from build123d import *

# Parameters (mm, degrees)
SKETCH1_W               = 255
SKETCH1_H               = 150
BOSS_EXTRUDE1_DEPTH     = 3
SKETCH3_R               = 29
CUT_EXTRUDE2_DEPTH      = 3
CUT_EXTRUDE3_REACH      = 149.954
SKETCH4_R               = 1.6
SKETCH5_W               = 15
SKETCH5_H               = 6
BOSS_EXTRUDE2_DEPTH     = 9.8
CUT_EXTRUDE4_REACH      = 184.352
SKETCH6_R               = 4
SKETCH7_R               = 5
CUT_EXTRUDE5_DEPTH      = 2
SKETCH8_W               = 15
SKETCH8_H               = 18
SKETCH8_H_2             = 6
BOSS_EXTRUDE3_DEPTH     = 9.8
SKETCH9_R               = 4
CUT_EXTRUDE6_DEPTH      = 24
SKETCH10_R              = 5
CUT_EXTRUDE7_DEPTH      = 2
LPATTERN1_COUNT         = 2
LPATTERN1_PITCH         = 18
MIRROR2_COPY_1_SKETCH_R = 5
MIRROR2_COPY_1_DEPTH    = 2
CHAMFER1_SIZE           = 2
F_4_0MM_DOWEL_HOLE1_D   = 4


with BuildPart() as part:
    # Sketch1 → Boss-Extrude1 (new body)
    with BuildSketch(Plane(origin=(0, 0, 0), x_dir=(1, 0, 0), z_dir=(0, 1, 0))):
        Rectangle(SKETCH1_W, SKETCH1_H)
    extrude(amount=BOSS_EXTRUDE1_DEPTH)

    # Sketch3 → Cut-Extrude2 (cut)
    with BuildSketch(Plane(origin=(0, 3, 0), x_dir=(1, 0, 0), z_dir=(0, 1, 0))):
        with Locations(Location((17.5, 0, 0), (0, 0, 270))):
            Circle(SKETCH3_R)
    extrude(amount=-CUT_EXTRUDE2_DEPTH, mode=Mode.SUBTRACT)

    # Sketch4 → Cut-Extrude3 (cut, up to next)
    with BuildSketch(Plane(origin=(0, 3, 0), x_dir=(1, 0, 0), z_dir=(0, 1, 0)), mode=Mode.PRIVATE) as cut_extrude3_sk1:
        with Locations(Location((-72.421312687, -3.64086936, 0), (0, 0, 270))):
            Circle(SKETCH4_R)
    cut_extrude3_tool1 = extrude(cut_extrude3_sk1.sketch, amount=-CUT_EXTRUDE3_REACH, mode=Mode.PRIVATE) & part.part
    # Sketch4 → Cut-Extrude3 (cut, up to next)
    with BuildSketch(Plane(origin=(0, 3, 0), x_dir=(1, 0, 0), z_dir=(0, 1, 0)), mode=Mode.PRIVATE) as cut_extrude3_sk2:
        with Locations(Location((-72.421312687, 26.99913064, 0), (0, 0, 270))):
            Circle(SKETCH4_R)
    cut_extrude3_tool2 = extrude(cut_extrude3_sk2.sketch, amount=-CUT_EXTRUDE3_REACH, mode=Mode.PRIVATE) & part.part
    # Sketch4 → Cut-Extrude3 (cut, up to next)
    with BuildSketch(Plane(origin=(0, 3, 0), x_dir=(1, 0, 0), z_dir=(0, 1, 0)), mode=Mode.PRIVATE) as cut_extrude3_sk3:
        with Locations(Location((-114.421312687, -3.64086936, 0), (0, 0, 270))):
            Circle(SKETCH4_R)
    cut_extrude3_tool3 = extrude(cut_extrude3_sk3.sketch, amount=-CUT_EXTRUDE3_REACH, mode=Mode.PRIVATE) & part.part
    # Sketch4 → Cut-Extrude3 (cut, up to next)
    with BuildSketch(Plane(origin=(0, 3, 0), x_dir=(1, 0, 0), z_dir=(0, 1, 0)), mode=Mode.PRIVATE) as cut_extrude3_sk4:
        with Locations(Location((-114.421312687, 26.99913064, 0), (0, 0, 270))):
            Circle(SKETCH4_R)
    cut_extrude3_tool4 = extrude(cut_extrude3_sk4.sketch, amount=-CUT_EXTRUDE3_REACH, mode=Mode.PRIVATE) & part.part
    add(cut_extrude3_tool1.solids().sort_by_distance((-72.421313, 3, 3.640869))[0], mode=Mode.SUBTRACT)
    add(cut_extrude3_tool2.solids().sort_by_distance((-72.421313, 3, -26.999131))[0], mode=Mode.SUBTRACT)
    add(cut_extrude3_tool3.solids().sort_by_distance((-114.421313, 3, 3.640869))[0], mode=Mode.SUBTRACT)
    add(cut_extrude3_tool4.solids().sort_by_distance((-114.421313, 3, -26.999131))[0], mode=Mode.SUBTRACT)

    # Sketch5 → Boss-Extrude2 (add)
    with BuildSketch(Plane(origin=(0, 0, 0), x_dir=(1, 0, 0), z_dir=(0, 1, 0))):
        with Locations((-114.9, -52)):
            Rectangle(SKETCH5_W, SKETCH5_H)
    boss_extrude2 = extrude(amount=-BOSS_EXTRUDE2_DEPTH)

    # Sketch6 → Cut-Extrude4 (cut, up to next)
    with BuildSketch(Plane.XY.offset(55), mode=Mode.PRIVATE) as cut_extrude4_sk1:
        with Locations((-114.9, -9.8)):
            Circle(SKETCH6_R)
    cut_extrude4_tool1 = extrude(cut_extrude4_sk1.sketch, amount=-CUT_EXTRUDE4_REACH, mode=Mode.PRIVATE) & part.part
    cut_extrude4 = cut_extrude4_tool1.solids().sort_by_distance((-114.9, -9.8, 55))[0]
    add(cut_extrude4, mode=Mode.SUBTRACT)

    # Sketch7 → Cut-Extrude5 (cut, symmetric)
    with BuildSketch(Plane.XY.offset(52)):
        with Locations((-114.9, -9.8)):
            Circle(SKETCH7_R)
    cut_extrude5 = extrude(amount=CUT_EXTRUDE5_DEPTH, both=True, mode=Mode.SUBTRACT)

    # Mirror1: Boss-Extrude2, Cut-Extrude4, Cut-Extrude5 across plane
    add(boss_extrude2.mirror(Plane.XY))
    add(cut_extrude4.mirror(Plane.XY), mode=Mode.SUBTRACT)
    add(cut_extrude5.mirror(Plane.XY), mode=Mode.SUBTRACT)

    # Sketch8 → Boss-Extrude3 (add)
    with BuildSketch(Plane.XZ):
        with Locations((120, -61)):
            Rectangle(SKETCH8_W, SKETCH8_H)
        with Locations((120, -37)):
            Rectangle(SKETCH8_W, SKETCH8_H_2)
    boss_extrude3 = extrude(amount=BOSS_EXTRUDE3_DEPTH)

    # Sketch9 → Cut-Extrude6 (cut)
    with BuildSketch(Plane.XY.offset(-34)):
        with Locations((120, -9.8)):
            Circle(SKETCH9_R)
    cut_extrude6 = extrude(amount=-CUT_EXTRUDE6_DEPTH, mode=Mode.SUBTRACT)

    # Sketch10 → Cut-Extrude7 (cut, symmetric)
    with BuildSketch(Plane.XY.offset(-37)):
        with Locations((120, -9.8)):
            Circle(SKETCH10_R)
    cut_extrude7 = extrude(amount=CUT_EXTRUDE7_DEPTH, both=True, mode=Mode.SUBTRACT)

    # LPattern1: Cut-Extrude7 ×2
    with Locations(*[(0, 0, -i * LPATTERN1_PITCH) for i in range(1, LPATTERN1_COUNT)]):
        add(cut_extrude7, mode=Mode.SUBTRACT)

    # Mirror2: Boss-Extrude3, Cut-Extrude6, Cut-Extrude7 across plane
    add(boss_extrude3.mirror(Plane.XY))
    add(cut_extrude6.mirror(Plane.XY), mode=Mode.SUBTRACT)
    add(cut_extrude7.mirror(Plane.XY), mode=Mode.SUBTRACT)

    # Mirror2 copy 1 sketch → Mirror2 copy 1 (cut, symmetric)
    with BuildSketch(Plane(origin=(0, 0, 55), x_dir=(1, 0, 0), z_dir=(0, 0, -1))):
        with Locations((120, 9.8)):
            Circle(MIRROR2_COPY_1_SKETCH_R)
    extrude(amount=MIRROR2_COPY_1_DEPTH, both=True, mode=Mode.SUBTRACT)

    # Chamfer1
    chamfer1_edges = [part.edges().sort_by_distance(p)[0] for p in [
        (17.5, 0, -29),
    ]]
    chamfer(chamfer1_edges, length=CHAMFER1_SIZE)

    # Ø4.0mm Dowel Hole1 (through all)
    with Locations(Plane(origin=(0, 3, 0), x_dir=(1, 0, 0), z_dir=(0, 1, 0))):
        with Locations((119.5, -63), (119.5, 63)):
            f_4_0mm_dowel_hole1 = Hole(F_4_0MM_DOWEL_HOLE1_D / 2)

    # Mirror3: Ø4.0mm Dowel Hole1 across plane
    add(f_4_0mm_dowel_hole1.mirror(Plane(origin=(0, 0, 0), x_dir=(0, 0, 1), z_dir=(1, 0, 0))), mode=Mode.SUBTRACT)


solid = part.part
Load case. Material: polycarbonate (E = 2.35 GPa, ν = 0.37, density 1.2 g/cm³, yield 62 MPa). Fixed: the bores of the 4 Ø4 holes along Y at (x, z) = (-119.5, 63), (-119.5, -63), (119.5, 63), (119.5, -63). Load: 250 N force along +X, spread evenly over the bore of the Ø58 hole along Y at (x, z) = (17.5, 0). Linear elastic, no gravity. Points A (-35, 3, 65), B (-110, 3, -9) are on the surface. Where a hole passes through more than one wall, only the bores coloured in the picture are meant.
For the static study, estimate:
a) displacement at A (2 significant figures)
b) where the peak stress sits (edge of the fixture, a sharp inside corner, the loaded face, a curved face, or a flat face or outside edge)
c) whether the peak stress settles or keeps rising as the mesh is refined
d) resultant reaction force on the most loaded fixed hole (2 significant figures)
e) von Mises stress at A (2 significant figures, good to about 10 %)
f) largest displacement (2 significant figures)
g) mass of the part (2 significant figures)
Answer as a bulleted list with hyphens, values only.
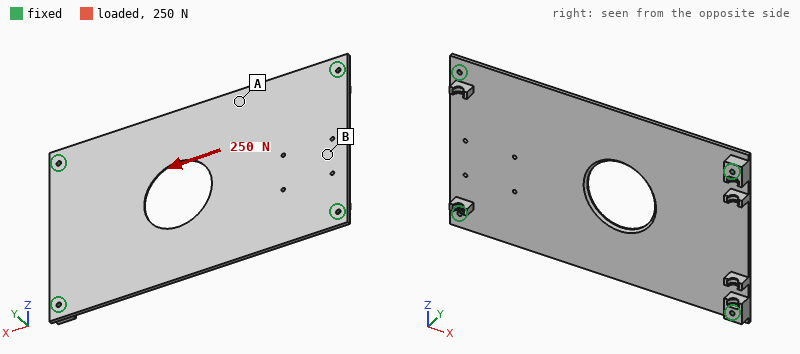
- 0.14 mm
- edge of the fixture
- keeps rising
- 75 N
- 0.38 MPa
- 0.17 mm
- 140 g
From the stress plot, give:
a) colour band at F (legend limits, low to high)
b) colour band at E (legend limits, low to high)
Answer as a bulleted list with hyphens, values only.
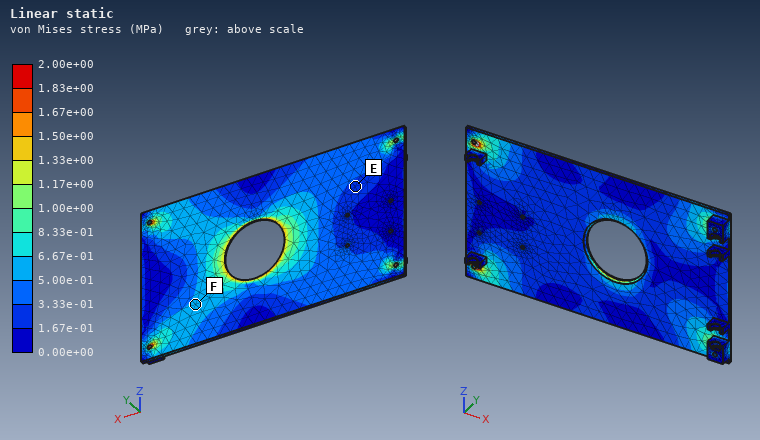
- 5.00e-01 to 6.67e-01 MPa
- 1.67e-01 to 3.33e-01 MPa
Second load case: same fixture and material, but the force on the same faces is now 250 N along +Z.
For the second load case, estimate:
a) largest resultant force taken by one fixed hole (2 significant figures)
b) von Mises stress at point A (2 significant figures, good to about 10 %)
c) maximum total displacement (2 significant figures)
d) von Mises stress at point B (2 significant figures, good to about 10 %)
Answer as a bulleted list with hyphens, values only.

- 90 N
- 0.38 MPa
- 0.33 mm
- 0.39 MPa
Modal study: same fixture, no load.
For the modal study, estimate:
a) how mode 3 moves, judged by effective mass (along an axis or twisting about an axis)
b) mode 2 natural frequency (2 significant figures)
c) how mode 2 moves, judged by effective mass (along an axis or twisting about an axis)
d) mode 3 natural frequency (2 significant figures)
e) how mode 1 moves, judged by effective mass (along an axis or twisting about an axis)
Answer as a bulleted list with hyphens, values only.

- twisting about Z
- 110 Hz
- twisting about X
- 180 Hz
- along Y
